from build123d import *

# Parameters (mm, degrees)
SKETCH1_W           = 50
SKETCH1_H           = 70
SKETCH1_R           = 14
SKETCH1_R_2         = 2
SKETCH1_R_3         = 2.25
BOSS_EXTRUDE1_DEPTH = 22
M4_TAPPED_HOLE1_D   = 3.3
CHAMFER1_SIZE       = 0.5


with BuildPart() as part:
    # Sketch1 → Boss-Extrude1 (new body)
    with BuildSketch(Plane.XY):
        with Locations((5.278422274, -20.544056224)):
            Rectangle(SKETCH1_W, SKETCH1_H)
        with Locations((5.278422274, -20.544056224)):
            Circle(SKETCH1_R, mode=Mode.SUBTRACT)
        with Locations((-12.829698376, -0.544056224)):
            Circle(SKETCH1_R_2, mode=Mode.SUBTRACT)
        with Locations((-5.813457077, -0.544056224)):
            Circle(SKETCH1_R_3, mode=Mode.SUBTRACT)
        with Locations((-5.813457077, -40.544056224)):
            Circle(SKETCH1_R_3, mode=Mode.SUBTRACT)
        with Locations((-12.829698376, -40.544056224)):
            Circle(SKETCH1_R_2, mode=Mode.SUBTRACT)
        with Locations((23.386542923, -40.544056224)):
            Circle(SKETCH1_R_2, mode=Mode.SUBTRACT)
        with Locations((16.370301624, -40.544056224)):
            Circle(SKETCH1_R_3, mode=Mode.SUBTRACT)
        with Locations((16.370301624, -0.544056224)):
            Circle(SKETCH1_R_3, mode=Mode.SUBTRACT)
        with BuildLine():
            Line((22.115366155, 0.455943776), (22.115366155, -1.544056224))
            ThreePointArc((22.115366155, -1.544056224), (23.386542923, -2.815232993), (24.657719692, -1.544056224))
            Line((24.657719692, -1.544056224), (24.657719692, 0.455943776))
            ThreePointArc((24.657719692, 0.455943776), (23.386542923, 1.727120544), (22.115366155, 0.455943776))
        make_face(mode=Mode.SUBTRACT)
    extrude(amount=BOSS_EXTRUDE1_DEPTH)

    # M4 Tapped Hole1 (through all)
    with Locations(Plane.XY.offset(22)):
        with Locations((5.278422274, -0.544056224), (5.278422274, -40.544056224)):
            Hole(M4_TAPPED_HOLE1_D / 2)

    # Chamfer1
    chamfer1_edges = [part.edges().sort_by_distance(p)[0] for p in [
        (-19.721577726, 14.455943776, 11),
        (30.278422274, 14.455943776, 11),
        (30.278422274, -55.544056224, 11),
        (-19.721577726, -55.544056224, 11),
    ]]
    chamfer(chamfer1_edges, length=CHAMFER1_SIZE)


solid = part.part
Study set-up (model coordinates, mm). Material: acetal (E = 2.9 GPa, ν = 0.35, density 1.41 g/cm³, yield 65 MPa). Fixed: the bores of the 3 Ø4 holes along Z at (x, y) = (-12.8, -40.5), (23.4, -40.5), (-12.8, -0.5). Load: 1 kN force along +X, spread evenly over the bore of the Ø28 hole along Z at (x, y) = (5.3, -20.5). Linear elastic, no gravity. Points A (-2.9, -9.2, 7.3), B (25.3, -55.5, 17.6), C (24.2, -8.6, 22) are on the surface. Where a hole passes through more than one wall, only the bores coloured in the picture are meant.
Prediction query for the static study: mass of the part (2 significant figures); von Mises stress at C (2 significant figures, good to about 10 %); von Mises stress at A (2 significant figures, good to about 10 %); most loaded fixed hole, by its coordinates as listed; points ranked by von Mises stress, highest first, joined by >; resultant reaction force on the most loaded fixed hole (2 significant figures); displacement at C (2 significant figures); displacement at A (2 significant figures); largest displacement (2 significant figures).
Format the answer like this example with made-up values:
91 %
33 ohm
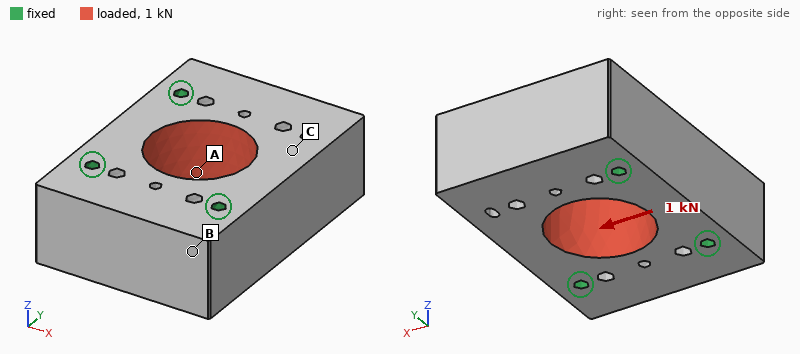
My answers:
85 g
0.75 MPa
1.3 MPa
(-12.8, -0.5)
A > C > B
470 N
16 µm
8.4 µm
19 µm
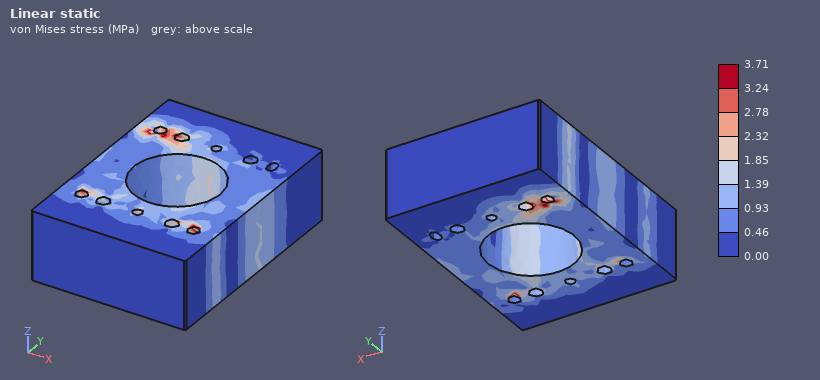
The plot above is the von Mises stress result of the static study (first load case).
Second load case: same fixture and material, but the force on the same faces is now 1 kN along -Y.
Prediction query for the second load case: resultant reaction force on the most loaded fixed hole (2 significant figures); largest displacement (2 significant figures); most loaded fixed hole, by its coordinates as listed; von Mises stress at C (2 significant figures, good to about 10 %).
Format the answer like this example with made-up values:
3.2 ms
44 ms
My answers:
460 N
14 µm
(23.4, -40.5)
0.44 MPa
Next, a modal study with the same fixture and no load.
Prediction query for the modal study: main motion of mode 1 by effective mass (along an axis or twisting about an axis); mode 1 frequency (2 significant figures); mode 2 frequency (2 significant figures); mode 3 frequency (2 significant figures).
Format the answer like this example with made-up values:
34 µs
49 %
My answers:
along Z
2500 Hz
4700 Hz
6200 Hz
